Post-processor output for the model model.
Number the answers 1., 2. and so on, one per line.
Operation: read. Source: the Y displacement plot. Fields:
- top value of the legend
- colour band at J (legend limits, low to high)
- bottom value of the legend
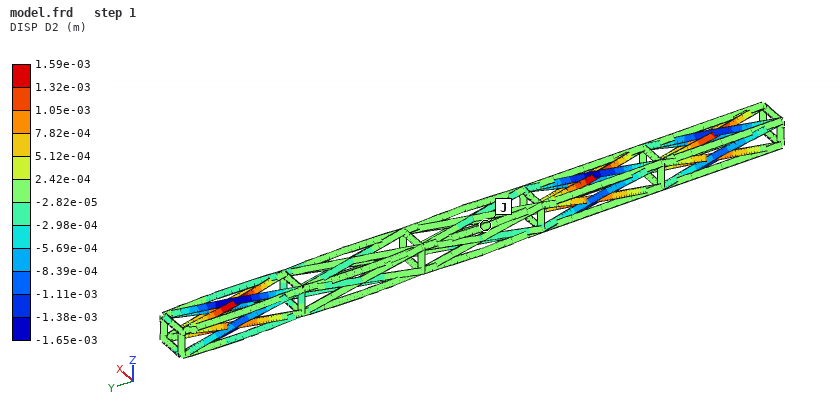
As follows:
1. 1.59e-03 m
2. -2.82e-05 to 2.42e-04 m
3. -1.65e-03 m
